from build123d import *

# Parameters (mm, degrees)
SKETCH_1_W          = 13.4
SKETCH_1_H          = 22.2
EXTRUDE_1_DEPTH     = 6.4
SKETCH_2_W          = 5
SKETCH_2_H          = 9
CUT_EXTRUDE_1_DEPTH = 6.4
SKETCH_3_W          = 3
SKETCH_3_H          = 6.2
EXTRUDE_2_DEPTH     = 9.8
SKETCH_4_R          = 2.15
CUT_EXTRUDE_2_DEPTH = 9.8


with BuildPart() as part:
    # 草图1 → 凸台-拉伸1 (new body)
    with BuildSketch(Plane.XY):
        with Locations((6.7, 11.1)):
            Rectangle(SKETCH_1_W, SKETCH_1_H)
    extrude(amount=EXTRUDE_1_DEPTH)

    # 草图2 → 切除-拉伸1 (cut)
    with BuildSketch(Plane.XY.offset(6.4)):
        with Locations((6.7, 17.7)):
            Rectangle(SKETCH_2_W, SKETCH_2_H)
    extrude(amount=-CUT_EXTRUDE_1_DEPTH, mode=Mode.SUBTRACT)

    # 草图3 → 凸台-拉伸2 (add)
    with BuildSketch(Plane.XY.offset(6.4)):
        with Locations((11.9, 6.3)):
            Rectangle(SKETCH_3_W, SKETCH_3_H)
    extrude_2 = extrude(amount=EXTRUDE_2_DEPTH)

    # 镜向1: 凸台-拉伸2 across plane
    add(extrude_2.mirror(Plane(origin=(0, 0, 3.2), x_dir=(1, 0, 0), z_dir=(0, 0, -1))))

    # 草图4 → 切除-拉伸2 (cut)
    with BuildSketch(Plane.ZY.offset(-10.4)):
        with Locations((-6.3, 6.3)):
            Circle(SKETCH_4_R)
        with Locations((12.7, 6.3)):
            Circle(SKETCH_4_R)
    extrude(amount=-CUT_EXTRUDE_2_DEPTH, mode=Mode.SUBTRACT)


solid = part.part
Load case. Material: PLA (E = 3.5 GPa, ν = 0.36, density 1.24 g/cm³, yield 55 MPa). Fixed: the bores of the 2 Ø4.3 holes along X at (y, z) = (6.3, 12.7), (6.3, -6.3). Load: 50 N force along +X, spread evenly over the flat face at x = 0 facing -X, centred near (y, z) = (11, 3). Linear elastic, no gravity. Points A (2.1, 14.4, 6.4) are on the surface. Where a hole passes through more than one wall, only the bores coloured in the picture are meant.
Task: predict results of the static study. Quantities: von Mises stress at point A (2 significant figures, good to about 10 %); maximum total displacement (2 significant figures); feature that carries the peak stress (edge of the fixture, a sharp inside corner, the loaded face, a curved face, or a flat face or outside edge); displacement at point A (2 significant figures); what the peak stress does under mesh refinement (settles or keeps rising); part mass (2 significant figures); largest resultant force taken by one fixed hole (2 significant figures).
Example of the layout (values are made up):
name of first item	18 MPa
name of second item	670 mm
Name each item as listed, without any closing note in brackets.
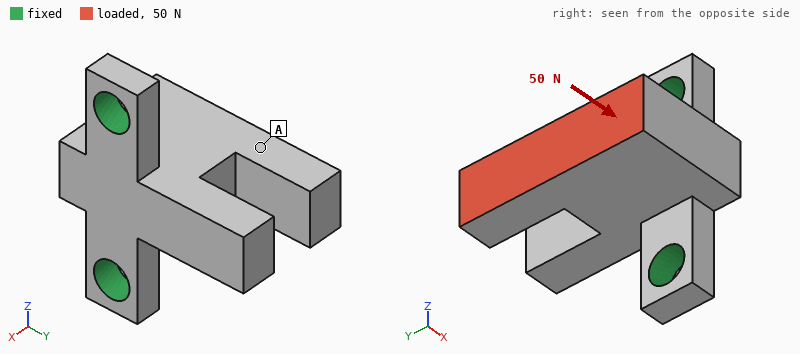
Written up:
von Mises stress at point A	1.8 MPa
maximum total displacement	0.27 mm
feature that carries the peak stress	edge of the fixture
displacement at point A	0.16 mm
what the peak stress does under mesh refinement	keeps rising
part mass	2.3 g
largest resultant force taken by one fixed hole	26 N
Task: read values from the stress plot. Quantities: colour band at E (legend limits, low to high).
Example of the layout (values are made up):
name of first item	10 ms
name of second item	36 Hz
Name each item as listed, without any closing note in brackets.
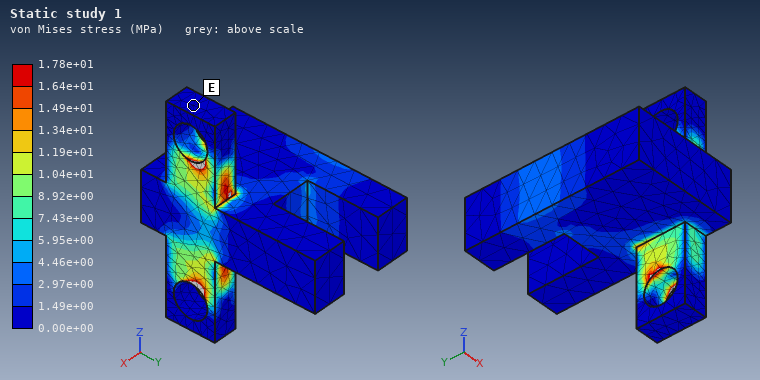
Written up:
colour band at E	0.00e+00 to 1.49e+00 MPa
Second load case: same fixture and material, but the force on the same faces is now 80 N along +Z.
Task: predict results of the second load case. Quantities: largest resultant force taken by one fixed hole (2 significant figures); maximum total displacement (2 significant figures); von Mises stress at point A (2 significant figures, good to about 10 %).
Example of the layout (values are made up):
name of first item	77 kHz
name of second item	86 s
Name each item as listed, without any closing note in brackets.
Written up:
largest resultant force taken by one fixed hole	94 N
maximum total displacement	0.26 mm
von Mises stress at point A	4.9 MPa
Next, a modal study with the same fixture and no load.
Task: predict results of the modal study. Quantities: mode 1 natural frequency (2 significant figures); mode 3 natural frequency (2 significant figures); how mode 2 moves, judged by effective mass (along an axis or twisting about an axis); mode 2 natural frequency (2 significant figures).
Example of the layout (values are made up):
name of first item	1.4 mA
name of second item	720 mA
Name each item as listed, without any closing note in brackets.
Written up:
mode 1 natural frequency	1700 Hz
mode 3 natural frequency	6200 Hz
how mode 2 moves, judged by effective mass	along Z
mode 2 natural frequency	4000 Hz
